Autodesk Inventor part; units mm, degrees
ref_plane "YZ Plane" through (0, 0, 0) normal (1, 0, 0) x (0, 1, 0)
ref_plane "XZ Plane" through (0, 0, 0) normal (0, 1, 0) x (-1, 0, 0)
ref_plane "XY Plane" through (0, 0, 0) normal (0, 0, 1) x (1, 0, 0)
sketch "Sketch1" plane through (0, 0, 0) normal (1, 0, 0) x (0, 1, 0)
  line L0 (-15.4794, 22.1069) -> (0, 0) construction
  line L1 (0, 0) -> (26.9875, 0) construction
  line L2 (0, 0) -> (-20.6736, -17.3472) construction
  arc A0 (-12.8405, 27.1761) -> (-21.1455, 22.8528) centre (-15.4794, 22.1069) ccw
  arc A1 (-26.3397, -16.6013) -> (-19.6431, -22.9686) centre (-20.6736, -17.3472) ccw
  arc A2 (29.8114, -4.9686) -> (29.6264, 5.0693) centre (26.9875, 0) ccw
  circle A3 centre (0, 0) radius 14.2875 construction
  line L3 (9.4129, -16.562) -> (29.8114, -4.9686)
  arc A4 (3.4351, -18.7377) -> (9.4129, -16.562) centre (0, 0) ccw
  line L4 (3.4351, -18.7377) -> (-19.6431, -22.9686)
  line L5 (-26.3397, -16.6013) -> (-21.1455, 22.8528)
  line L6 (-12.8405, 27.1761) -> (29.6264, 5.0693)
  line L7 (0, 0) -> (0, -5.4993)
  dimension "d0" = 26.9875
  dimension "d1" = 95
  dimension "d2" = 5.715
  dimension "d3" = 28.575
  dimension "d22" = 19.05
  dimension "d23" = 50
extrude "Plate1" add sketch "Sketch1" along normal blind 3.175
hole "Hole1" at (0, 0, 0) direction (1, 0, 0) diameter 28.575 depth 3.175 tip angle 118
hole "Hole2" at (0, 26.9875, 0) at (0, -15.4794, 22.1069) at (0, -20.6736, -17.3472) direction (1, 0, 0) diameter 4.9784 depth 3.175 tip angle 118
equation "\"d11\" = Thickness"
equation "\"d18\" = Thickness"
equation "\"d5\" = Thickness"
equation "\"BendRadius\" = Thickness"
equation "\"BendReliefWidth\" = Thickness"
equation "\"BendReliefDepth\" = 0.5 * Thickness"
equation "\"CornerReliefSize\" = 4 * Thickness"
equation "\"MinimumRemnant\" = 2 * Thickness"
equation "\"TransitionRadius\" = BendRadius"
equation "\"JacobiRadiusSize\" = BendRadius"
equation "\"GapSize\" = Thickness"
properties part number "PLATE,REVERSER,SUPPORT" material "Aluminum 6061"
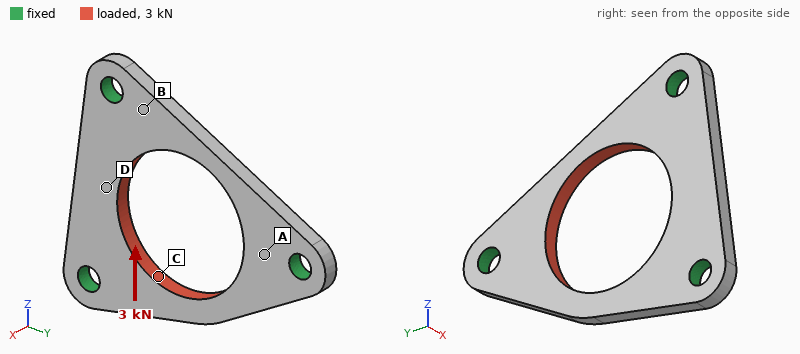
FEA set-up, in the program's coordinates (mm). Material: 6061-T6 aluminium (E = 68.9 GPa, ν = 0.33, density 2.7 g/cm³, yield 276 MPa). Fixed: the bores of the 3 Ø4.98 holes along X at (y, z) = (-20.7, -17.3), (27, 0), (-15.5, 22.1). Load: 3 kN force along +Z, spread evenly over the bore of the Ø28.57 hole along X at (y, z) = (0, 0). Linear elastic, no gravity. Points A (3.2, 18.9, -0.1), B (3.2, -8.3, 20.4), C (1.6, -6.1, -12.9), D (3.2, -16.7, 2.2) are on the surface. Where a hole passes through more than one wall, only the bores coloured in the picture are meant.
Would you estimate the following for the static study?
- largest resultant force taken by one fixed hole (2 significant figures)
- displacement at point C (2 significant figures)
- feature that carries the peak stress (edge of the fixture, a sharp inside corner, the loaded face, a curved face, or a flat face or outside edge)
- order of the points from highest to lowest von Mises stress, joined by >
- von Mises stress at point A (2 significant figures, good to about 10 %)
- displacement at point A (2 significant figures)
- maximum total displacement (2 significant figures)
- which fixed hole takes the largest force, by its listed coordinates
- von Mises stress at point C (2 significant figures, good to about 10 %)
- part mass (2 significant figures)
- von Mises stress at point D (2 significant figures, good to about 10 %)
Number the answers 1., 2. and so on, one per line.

1. 1.4 kN
2. 17 µm
3. edge of the fixture
4. C > A > D > B
5. 46 MPa
6. 15 µm
7. 37 µm
8. (27, 0)
9. 62 MPa
10. 10 g
11. 27 MPa
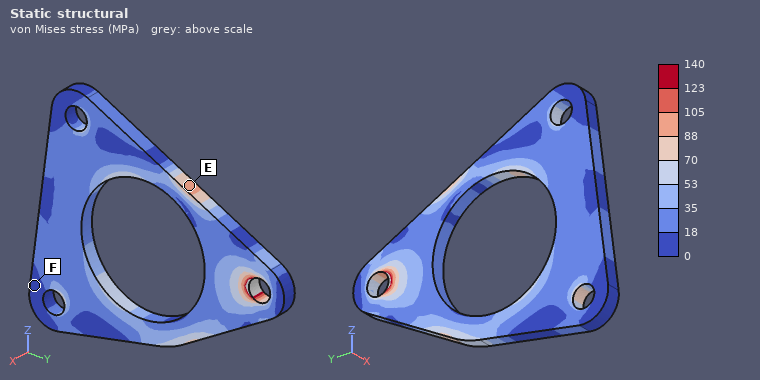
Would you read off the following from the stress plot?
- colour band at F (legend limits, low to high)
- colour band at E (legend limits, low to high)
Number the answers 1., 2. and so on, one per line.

1. 0 to 18 MPa
2. 88 to 105 MPa
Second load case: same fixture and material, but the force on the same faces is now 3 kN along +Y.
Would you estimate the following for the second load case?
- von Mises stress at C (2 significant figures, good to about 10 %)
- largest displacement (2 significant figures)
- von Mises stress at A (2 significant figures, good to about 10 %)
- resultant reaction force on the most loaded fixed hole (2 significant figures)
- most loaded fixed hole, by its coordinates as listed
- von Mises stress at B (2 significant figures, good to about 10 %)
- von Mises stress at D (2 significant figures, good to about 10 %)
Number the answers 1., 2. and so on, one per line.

1. 18 MPa
2. 19 µm
3. 16 MPa
4. 1.2 kN
5. (-20.7, -17.3)
6. 27 MPa
7. 14 MPa
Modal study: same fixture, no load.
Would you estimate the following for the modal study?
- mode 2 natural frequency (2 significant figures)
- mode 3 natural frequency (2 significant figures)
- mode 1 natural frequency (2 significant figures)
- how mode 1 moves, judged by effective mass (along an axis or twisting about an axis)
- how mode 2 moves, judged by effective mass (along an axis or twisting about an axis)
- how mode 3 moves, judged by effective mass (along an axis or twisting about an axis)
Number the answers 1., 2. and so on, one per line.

1. 10000 Hz
2. 12 kHz
3. 8000 Hz
4. along X
5. along X
6. along X
